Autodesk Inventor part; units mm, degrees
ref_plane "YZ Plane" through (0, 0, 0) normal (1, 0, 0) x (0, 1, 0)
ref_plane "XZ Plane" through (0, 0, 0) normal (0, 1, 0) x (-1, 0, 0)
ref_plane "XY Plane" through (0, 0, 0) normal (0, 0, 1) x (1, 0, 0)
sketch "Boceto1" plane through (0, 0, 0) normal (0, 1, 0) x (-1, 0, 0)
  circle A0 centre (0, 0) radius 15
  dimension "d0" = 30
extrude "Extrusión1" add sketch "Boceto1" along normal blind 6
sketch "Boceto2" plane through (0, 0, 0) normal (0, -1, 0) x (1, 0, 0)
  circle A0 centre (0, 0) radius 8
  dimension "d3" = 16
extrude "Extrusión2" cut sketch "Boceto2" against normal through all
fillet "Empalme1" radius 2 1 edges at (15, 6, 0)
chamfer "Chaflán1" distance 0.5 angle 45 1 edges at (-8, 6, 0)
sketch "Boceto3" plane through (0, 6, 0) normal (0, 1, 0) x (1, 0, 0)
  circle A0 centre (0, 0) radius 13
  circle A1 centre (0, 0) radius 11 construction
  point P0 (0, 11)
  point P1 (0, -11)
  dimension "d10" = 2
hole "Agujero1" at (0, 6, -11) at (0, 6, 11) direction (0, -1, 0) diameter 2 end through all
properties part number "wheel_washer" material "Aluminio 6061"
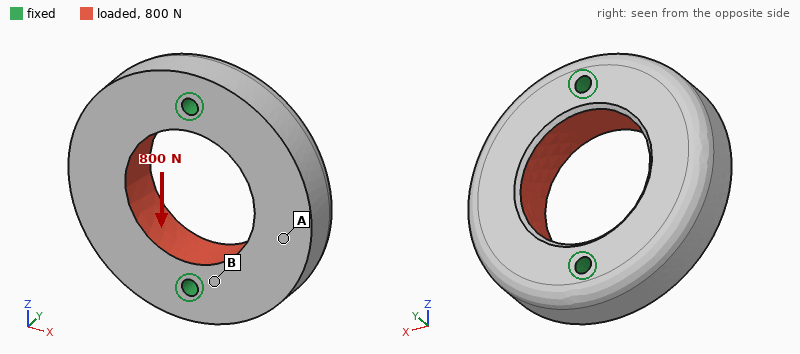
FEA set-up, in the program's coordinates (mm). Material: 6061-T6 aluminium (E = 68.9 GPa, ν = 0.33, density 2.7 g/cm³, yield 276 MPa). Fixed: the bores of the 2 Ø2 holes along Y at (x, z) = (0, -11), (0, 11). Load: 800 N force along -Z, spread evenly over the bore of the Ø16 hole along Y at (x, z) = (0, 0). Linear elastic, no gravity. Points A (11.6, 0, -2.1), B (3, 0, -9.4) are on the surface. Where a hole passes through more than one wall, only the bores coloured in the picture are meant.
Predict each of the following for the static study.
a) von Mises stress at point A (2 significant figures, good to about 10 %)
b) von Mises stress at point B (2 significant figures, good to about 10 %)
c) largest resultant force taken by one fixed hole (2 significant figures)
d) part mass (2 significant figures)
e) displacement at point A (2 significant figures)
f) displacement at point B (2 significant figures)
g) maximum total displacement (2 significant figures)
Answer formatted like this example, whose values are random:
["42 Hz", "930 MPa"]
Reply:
["3.2 MPa", "10 MPa", "400 N", "7.9 g", "1.9 µm", "0.80 µm", "2.4 µm"]
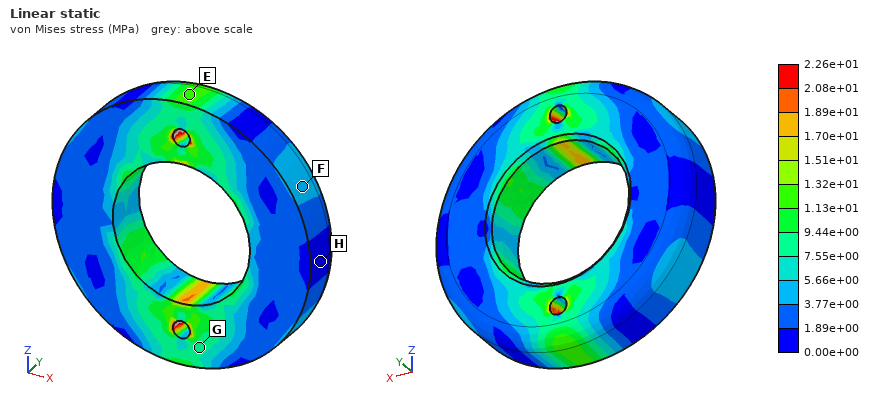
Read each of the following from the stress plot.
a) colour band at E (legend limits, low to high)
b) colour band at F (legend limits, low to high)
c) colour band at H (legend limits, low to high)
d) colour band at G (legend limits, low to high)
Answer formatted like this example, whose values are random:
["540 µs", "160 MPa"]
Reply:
["1.13e+01 to 1.32e+01 MPa", "3.77e+00 to 5.66e+00 MPa", "0.00e+00 to 1.89e+00 MPa", "7.55e+00 to 9.44e+00 MPa"]
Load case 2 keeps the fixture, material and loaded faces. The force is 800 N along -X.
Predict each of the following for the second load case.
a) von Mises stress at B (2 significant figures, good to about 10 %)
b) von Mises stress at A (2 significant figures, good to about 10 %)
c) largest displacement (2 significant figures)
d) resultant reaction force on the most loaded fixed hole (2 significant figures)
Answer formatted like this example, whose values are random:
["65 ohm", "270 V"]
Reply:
["9.5 MPa", "3.7 MPa", "1.8 µm", "400 N"]
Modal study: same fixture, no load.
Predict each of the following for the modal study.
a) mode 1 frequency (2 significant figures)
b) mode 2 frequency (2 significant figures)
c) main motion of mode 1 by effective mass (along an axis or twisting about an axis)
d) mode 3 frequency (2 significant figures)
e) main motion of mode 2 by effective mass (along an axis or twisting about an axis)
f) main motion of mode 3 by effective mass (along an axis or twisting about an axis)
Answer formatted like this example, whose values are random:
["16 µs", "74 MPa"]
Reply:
["16 kHz", "17 kHz", "twisting about Z", "28 kHz", "along Y", "twisting about Y"]
